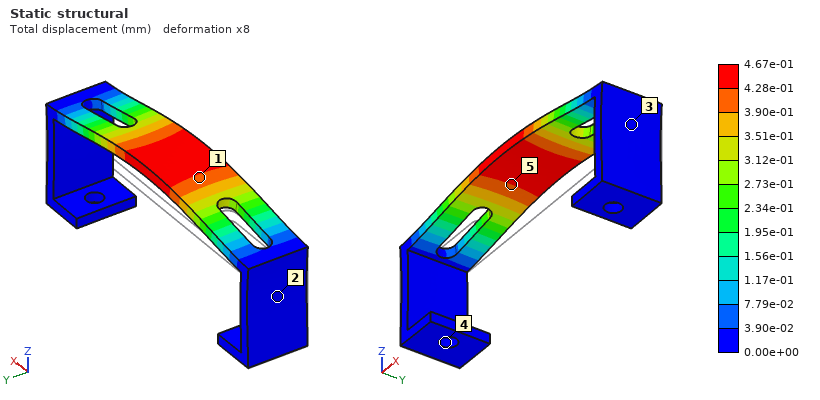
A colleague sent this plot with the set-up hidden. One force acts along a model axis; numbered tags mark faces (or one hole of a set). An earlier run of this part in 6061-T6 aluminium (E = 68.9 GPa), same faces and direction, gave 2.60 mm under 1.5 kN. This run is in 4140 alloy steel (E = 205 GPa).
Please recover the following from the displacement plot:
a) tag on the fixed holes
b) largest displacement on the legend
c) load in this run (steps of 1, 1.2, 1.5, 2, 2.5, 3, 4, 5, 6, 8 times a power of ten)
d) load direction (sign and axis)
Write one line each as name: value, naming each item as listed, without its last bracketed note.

tag on the fixed holes: 4
largest displacement on the legend: 4.67e-01 mm
load in this run: 800 N
load direction: +Z
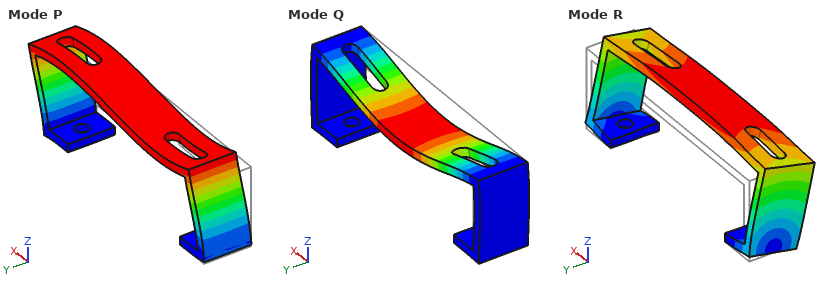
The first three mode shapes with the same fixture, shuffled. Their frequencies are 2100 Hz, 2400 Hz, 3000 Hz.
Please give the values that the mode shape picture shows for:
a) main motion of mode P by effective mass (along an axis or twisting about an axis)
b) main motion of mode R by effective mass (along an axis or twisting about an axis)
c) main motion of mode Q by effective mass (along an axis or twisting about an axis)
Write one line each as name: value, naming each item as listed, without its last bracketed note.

main motion of mode P by effective mass: along X
main motion of mode R by effective mass: along Y
main motion of mode Q by effective mass: along Z
